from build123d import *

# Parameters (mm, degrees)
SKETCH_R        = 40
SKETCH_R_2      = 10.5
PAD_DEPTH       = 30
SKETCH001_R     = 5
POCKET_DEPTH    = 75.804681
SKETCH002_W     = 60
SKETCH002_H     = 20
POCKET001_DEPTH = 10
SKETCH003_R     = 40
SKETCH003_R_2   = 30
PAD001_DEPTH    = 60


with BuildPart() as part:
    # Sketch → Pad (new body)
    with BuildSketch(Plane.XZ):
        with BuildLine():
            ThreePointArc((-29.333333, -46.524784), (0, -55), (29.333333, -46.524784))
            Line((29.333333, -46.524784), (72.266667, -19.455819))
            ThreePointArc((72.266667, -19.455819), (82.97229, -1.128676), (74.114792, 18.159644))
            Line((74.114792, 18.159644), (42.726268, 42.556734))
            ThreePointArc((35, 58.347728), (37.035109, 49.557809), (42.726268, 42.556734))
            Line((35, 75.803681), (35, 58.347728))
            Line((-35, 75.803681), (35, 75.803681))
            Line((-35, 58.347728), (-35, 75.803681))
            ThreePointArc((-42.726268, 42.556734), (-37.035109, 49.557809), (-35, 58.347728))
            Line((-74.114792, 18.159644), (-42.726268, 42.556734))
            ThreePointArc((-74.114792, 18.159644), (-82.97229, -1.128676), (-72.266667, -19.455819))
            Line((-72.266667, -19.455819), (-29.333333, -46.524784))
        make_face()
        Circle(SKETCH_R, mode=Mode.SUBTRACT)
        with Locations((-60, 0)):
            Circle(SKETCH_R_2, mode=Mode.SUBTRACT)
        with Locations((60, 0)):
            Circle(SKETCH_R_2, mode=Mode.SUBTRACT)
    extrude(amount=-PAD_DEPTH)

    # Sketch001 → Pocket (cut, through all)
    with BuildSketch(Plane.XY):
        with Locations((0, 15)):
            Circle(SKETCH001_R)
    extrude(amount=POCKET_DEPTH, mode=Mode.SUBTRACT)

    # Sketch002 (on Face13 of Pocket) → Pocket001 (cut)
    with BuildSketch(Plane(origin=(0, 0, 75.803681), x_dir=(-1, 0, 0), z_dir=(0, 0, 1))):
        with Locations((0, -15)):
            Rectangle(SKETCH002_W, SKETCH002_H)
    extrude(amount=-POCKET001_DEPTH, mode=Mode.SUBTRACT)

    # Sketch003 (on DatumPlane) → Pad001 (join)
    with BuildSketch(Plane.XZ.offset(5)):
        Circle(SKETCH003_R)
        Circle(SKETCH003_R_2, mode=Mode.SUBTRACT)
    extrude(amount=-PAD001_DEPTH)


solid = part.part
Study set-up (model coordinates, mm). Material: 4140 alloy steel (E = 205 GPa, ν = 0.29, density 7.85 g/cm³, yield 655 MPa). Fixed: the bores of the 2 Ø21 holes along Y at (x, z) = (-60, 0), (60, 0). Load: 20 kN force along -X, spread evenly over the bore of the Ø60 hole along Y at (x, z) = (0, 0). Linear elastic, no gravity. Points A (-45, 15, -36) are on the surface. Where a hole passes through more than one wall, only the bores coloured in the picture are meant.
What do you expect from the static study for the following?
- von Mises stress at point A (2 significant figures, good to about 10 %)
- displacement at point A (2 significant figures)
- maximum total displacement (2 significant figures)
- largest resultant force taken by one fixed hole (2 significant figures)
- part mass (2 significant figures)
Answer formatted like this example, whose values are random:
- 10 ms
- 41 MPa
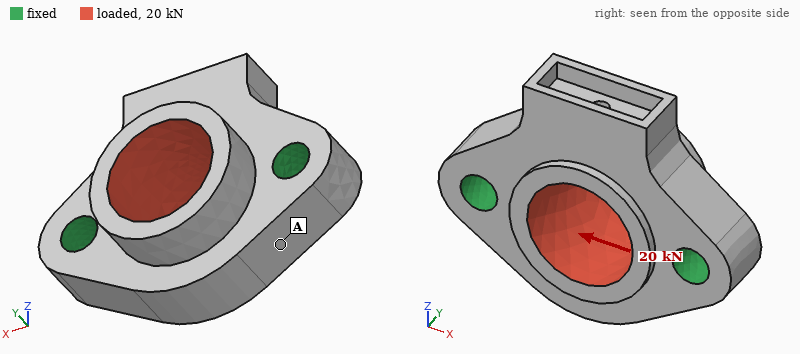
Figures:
- 2.2 MPa
- 1.3 µm
- 3.8 µm
- 10 kN
- 3.0 kg
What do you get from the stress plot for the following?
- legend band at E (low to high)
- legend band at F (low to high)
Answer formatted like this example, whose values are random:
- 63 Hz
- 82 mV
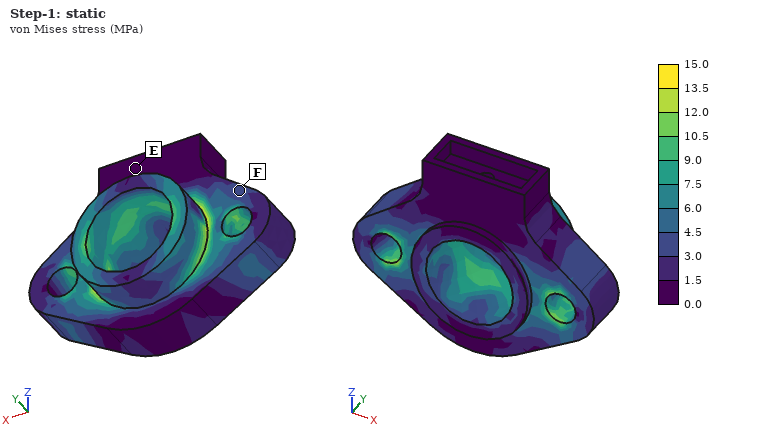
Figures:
- 0.0 to 1.5 MPa
- 3.0 to 4.5 MPa
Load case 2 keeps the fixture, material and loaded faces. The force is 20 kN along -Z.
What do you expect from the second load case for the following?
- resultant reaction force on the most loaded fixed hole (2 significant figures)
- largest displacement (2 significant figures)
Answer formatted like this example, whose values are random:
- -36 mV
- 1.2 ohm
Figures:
- 10 kN
- 8.1 µm
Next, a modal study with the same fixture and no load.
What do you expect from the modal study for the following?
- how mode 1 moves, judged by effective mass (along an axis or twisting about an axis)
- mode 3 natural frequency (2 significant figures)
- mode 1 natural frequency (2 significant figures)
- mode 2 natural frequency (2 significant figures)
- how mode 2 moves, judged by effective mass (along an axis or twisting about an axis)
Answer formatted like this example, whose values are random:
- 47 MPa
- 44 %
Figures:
- along Y
- 9300 Hz
- 4100 Hz
- 6100 Hz
- along Y
